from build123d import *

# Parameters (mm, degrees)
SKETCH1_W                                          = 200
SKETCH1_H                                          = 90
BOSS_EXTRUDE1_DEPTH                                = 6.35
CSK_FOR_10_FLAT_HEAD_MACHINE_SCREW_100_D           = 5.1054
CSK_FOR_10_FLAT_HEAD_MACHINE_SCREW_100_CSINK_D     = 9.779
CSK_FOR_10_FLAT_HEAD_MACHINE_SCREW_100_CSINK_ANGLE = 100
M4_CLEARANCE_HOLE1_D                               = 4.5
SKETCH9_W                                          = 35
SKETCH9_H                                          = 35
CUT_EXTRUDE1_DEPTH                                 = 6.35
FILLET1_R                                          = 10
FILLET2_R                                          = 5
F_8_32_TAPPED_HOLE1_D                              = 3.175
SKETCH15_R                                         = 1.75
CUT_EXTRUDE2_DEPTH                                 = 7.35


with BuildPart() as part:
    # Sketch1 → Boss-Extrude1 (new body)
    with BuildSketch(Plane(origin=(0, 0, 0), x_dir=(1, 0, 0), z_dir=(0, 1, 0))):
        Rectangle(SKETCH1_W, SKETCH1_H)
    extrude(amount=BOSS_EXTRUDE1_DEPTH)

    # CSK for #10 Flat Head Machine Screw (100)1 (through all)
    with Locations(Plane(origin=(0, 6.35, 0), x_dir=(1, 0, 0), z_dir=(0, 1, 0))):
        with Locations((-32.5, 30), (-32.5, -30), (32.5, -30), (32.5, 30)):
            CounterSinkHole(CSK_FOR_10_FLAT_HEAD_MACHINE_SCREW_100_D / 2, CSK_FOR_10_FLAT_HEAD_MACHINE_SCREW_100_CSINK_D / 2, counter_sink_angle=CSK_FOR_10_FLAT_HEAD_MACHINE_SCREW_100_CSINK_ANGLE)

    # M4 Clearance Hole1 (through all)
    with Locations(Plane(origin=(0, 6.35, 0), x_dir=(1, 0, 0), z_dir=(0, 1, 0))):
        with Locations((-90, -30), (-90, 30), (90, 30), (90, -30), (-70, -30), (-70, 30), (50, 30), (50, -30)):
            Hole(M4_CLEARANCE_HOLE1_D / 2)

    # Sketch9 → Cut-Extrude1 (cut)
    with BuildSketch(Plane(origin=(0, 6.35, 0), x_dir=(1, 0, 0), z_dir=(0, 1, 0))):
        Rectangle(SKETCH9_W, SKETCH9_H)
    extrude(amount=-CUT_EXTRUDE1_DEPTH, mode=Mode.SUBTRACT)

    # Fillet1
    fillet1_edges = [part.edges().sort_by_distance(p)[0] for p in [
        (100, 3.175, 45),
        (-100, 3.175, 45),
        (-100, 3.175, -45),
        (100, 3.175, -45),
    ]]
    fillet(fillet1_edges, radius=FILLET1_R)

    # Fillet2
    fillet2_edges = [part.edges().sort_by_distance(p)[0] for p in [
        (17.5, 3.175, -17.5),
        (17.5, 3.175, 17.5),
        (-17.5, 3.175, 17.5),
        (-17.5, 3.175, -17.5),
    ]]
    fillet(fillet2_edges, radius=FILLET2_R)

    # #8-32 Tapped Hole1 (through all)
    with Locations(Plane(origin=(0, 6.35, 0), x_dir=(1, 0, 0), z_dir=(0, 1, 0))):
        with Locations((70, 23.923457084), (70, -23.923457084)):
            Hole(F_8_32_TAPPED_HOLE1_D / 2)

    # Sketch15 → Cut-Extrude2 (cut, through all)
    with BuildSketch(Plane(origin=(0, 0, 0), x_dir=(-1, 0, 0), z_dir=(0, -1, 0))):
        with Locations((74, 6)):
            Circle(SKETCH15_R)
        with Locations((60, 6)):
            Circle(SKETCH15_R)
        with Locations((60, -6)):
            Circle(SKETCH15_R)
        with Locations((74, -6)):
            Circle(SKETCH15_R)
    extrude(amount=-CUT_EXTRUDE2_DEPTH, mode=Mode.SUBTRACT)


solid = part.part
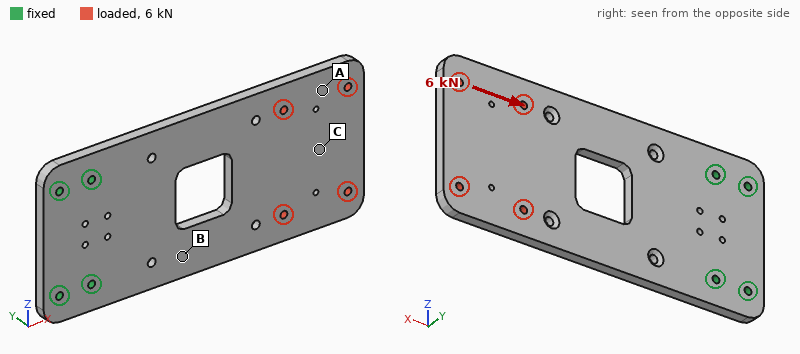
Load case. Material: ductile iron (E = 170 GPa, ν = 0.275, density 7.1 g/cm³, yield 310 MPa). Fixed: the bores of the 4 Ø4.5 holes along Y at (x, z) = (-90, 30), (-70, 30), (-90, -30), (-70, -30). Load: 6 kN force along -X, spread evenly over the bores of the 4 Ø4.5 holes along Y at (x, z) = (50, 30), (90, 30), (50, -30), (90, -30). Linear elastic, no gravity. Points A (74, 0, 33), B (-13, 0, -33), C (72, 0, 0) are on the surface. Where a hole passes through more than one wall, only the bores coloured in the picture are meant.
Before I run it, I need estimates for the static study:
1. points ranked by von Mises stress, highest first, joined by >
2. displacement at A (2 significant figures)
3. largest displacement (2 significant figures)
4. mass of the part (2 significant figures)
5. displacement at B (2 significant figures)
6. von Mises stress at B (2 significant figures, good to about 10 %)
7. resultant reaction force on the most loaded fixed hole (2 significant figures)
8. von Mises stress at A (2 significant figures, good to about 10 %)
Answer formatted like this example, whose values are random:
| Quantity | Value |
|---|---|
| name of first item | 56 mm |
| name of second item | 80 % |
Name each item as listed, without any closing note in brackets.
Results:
| Quantity | Value |
|---|---|
| points ranked by von Mises stress, highest first, joined by > | B > A > C |
| displacement at A | 13 µm |
| largest displacement | 15 µm |
| mass of the part | 740 g |
| displacement at B | 5.8 µm |
| von Mises stress at B | 15 MPa |
| resultant reaction force on the most loaded fixed hole | 2.2 kN |
| von Mises stress at A | 7.9 MPa |
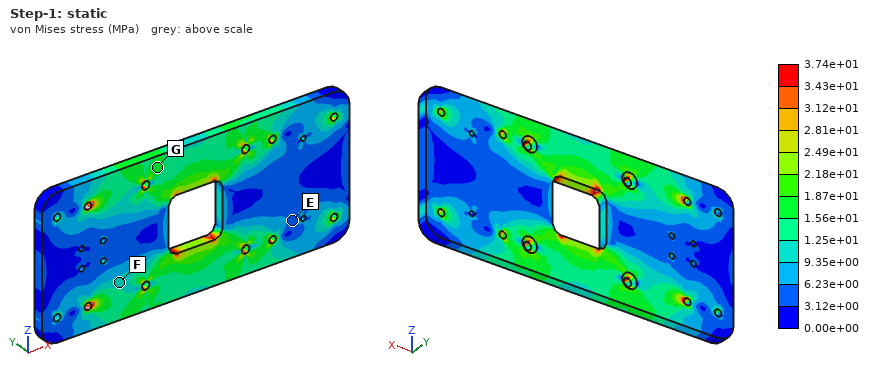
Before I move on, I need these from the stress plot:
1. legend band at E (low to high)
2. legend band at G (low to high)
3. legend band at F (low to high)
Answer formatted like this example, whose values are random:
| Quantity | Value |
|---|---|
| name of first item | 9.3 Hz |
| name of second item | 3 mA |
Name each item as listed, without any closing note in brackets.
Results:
| Quantity | Value |
|---|---|
| legend band at E | 3.12e+00 to 6.23e+00 MPa |
| legend band at G | 1.56e+01 to 1.87e+01 MPa |
| legend band at F | 9.35e+00 to 1.25e+01 MPa |
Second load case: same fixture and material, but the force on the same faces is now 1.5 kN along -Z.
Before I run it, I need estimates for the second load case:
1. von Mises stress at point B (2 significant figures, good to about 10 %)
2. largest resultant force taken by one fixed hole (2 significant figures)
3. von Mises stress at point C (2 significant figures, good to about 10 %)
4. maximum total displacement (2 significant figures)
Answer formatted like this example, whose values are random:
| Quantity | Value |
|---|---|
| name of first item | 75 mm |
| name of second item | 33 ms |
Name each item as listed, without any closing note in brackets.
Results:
| Quantity | Value |
|---|---|
| von Mises stress at point B | 15 MPa |
| largest resultant force taken by one fixed hole | 2.7 kN |
| von Mises stress at point C | 3.9 MPa |
| maximum total displacement | 49 µm |
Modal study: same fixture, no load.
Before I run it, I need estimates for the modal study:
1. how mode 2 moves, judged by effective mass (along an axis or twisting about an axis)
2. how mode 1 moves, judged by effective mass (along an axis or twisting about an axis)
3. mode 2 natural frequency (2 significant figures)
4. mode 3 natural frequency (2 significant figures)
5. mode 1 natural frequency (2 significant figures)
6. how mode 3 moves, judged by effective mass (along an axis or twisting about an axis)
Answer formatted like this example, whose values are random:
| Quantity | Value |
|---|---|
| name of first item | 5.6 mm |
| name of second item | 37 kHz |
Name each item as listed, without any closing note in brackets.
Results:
| Quantity | Value |
|---|---|
| how mode 2 moves, judged by effective mass | twisting about X |
| how mode 1 moves, judged by effective mass | along Y |
| mode 2 natural frequency | 650 Hz |
| mode 3 natural frequency | 1000 Hz |
| mode 1 natural frequency | 160 Hz |
| how mode 3 moves, judged by effective mass | along Y |
